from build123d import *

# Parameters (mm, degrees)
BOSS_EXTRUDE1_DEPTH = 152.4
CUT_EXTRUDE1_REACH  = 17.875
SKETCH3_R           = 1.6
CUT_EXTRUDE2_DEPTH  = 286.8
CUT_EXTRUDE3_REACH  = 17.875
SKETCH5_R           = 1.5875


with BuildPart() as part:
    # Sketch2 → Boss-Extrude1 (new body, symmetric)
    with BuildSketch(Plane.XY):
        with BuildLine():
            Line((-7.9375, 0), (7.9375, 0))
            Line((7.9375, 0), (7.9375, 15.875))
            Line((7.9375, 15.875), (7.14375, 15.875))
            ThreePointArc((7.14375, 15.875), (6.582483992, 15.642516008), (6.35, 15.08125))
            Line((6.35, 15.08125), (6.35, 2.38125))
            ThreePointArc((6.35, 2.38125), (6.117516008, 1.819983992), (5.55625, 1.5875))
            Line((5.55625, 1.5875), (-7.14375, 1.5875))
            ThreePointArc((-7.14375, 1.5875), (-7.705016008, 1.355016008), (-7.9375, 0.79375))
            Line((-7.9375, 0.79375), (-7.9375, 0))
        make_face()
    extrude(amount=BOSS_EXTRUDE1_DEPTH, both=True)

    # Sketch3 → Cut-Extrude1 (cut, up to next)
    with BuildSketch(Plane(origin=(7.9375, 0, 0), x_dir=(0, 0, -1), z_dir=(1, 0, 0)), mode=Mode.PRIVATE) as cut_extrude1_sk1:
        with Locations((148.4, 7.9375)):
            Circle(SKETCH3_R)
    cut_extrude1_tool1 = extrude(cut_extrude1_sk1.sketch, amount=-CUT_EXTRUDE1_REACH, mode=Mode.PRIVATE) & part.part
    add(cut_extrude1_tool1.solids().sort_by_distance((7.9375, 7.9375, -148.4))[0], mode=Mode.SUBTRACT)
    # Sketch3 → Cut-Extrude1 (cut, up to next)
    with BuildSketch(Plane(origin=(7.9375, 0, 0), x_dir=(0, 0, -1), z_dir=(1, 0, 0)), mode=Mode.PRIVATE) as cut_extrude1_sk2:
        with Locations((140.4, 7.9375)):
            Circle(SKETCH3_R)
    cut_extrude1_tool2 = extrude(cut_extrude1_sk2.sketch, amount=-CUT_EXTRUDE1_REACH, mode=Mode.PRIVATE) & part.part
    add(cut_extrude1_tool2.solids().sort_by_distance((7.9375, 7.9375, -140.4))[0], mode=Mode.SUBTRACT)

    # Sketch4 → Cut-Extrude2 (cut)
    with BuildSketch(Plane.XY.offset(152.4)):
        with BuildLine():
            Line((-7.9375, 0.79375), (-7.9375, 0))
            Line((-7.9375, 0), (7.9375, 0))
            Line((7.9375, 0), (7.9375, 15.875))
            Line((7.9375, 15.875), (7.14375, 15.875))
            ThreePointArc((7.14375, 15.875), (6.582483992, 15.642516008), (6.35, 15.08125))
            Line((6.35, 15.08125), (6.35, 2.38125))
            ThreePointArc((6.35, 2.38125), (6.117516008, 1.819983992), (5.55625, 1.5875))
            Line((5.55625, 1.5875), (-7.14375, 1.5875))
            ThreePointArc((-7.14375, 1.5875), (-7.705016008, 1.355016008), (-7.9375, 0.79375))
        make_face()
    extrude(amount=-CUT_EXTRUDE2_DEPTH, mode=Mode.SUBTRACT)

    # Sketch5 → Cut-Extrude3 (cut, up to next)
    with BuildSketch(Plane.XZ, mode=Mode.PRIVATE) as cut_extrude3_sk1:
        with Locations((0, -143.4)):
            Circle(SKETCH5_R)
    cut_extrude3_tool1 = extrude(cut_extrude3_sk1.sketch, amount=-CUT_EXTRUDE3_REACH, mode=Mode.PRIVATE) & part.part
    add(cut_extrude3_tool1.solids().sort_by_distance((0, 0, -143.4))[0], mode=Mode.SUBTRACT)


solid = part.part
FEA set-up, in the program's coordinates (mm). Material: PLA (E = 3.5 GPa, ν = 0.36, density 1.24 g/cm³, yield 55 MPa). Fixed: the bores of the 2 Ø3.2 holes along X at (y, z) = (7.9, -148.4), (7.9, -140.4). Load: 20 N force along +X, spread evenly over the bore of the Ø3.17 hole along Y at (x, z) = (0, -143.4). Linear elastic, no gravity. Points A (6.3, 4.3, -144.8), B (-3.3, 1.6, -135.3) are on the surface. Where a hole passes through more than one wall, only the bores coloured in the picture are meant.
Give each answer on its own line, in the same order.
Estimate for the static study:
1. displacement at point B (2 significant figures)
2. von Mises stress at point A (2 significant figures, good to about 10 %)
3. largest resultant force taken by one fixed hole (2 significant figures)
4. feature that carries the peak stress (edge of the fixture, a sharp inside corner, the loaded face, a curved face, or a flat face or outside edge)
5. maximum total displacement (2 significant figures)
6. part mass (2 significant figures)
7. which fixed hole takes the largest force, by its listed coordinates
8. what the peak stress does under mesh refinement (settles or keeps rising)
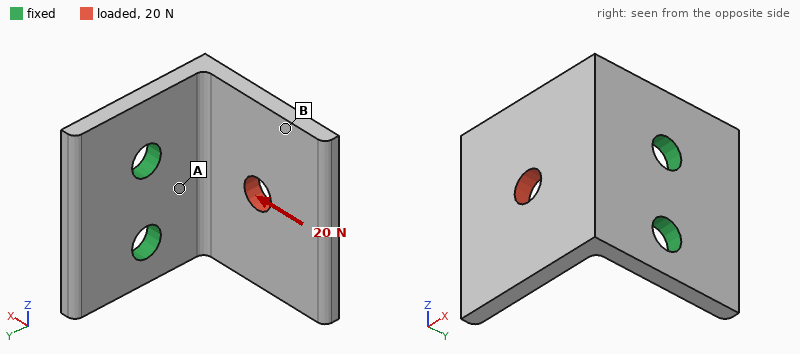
0.19 mm
8.0 MPa
12 N
edge of the fixture
0.28 mm
1.0 g
(7.9, -140.4)
keeps rising
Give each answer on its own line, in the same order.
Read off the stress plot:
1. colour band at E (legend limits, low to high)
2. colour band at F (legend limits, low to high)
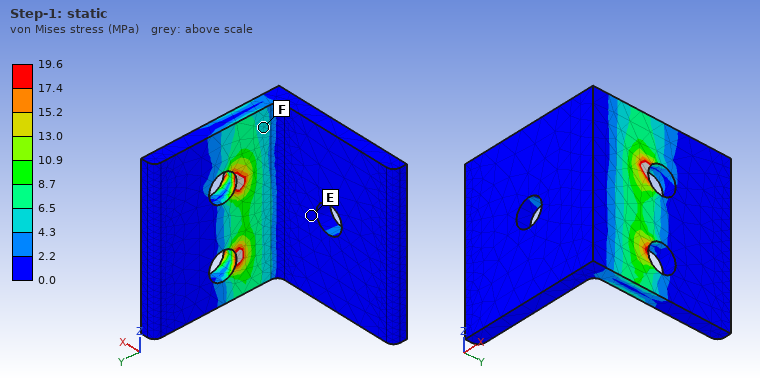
0.0 to 2.2 MPa
4.3 to 6.5 MPa
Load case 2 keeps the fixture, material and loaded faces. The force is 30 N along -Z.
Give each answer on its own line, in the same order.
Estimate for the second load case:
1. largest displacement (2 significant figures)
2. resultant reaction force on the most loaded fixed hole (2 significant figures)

0.27 mm
31 N
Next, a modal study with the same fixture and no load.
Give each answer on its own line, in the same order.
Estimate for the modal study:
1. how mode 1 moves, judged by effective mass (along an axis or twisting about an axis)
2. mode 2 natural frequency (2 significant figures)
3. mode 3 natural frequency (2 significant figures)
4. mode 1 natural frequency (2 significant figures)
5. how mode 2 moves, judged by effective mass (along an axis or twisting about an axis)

along Y
2500 Hz
3900 Hz
1300 Hz
along Z
